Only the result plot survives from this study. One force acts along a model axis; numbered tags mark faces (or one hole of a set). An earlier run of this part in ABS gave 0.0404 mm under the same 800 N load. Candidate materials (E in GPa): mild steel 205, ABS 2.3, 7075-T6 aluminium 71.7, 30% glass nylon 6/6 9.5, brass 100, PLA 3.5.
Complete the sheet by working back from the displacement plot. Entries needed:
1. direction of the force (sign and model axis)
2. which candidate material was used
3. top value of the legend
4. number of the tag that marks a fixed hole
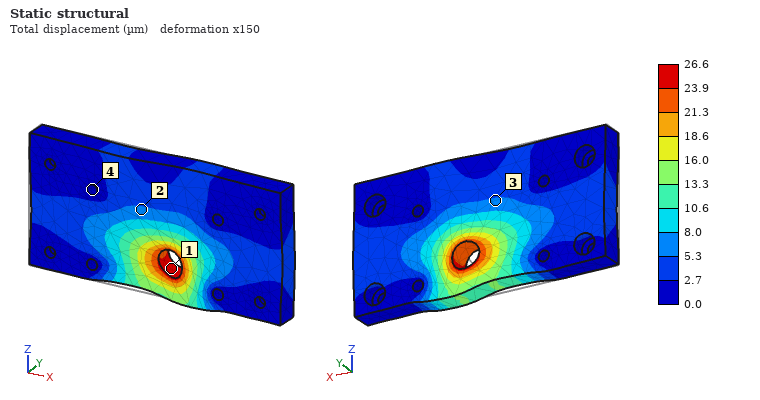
+X
PLA
26.6 µm
4
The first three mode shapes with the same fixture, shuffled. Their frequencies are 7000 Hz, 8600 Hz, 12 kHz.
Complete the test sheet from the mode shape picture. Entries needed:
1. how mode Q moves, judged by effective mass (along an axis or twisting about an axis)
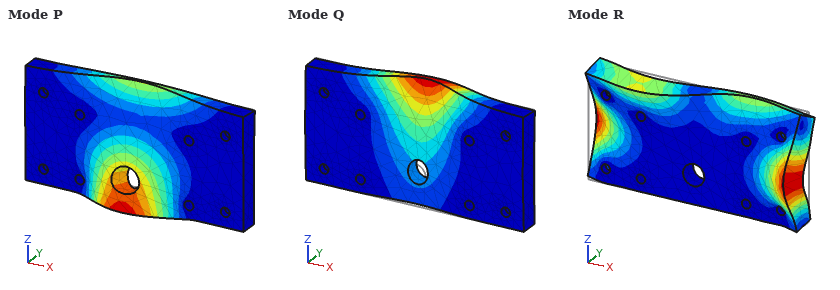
along Y
